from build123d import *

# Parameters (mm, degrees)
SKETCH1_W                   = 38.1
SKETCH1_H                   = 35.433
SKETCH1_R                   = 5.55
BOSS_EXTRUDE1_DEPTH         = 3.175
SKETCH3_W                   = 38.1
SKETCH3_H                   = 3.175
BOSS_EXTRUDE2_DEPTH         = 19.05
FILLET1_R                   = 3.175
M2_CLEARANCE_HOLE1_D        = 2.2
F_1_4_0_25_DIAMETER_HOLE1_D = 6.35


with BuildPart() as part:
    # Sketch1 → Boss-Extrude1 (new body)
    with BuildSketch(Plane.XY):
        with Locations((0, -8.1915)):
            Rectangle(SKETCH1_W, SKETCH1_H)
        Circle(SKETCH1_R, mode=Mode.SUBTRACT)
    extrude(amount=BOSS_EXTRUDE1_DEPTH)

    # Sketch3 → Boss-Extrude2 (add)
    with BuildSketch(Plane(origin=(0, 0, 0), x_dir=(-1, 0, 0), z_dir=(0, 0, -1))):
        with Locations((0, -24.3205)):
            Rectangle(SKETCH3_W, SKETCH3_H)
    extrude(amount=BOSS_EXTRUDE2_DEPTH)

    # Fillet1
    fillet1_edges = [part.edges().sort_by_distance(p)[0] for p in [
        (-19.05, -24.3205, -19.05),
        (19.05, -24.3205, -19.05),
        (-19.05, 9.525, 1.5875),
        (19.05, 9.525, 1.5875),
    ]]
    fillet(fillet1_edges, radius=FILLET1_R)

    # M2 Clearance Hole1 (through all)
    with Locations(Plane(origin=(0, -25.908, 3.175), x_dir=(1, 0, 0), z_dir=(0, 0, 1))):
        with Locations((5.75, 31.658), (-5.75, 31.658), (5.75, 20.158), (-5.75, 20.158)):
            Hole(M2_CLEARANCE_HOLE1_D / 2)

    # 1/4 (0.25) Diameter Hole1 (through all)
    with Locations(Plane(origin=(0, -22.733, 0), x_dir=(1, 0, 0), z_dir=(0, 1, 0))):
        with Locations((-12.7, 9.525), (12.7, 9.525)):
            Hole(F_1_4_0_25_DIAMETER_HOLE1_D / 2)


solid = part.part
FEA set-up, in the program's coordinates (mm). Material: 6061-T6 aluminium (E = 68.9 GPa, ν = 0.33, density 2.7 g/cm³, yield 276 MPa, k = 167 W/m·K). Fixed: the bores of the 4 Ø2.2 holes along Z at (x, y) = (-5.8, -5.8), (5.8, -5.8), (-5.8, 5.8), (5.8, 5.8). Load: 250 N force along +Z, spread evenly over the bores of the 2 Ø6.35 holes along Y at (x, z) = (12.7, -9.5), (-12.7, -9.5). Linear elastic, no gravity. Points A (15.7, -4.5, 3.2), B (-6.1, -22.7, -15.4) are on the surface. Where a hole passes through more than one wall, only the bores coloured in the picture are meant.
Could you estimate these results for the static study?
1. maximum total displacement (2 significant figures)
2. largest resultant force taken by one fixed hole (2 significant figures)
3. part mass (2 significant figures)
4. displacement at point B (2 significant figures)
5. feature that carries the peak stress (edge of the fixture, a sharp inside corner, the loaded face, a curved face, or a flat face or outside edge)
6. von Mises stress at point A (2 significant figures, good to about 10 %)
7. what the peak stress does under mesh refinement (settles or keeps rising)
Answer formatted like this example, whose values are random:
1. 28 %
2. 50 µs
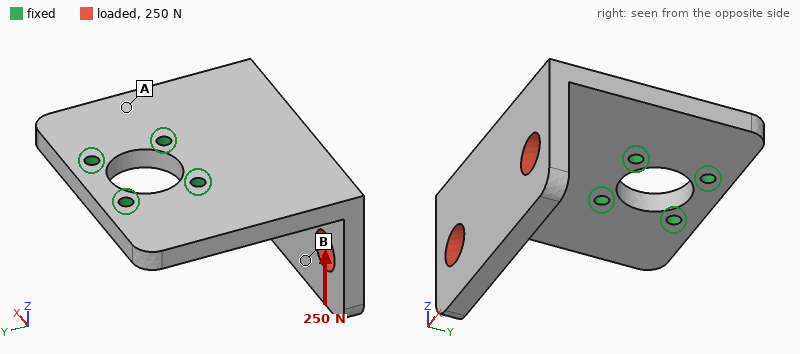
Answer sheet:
1. 0.17 mm
2. 190 N
3. 16 g
4. 0.14 mm
5. edge of the fixture
6. 33 MPa
7. keeps rising
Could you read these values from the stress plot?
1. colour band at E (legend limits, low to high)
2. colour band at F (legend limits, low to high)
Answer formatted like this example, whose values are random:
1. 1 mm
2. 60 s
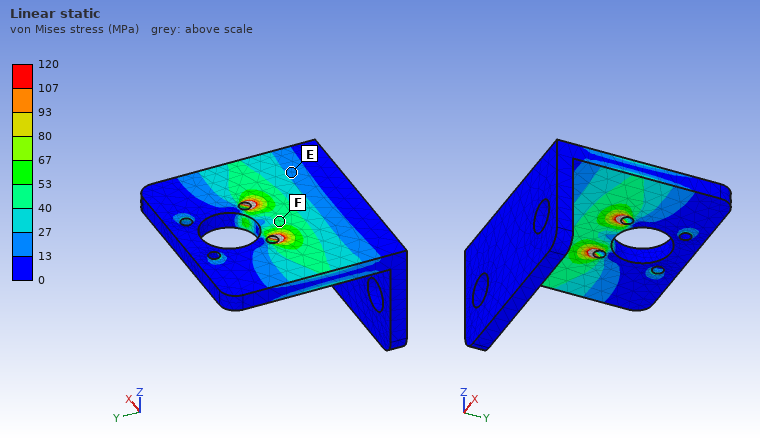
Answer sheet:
1. 13 to 27 MPa
2. 40 to 53 MPa
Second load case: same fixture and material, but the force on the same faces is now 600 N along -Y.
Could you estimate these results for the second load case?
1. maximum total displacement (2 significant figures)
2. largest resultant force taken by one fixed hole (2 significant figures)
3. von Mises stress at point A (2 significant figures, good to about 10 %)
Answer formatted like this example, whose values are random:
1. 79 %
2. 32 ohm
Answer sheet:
1. 0.49 mm
2. 280 N
3. 52 MPa
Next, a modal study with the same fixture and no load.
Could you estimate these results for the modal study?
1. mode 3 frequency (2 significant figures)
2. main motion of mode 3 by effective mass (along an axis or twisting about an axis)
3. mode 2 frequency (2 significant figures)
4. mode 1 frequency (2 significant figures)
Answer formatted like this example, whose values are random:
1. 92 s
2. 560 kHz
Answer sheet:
1. 6000 Hz
2. along Z
3. 3400 Hz
4. 2200 Hz
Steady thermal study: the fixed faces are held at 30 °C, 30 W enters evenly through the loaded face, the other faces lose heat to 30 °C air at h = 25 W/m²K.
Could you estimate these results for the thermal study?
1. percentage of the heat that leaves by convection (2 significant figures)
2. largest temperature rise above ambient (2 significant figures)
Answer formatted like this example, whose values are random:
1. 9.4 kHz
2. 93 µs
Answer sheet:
1. 8.2 %
2. 51 K
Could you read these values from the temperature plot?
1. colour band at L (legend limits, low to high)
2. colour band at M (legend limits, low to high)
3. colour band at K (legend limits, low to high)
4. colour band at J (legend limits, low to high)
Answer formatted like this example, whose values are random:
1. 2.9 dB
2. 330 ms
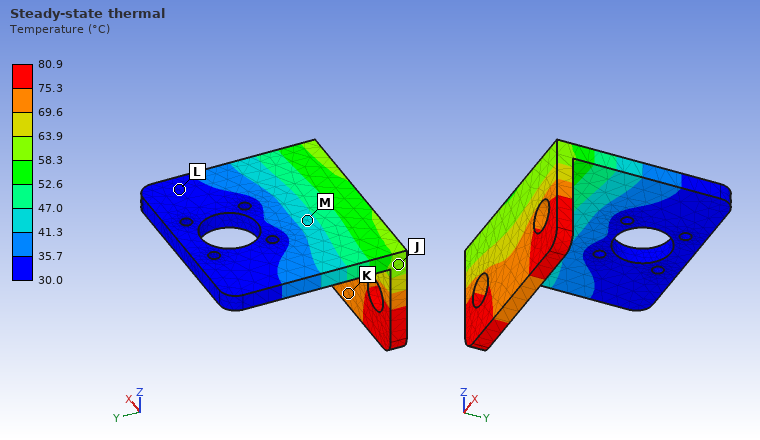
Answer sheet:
1. 30.0 to 35.7 °C
2. 41.3 to 47.0 °C
3. 69.6 to 75.3 °C
4. 58.3 to 63.9 °C
